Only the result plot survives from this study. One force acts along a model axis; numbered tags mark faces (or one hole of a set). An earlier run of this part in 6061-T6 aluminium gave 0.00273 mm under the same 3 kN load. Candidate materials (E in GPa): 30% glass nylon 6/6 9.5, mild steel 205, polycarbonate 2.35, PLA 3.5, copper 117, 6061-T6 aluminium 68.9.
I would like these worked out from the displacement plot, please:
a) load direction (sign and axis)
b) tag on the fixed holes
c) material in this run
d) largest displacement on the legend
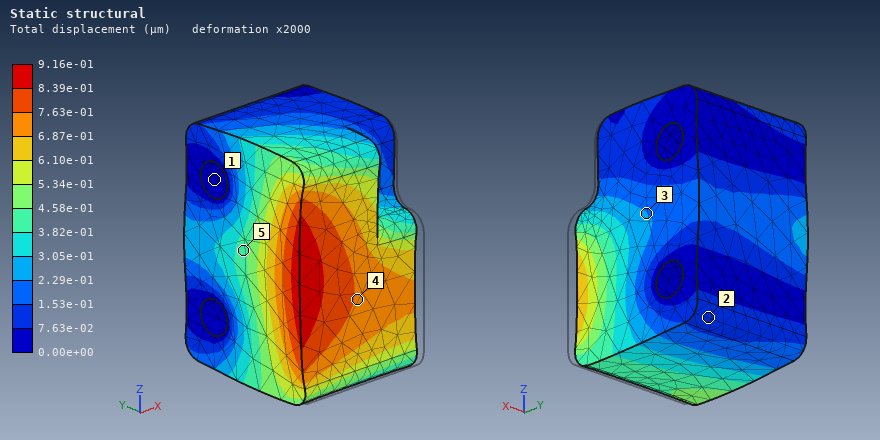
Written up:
+Y
1
mild steel
9.16e-01 µm
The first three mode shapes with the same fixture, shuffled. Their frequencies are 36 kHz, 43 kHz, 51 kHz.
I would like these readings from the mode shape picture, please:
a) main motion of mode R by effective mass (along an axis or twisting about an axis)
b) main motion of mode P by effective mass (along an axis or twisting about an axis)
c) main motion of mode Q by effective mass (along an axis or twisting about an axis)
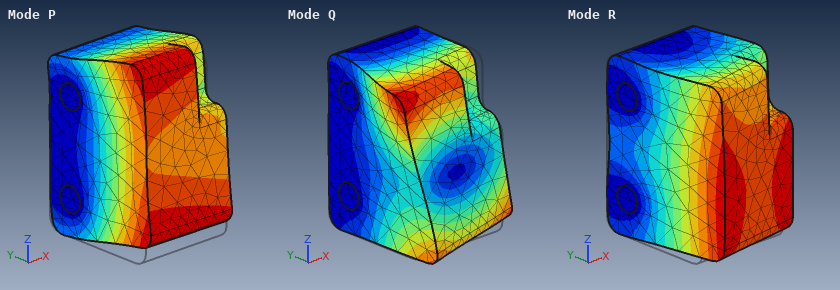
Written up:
along X
along Z
twisting about Y
